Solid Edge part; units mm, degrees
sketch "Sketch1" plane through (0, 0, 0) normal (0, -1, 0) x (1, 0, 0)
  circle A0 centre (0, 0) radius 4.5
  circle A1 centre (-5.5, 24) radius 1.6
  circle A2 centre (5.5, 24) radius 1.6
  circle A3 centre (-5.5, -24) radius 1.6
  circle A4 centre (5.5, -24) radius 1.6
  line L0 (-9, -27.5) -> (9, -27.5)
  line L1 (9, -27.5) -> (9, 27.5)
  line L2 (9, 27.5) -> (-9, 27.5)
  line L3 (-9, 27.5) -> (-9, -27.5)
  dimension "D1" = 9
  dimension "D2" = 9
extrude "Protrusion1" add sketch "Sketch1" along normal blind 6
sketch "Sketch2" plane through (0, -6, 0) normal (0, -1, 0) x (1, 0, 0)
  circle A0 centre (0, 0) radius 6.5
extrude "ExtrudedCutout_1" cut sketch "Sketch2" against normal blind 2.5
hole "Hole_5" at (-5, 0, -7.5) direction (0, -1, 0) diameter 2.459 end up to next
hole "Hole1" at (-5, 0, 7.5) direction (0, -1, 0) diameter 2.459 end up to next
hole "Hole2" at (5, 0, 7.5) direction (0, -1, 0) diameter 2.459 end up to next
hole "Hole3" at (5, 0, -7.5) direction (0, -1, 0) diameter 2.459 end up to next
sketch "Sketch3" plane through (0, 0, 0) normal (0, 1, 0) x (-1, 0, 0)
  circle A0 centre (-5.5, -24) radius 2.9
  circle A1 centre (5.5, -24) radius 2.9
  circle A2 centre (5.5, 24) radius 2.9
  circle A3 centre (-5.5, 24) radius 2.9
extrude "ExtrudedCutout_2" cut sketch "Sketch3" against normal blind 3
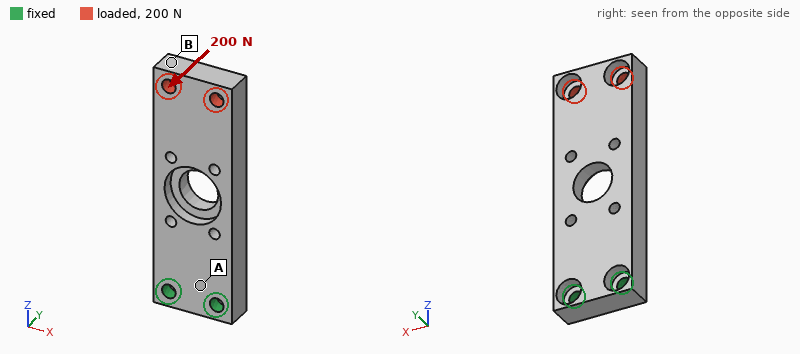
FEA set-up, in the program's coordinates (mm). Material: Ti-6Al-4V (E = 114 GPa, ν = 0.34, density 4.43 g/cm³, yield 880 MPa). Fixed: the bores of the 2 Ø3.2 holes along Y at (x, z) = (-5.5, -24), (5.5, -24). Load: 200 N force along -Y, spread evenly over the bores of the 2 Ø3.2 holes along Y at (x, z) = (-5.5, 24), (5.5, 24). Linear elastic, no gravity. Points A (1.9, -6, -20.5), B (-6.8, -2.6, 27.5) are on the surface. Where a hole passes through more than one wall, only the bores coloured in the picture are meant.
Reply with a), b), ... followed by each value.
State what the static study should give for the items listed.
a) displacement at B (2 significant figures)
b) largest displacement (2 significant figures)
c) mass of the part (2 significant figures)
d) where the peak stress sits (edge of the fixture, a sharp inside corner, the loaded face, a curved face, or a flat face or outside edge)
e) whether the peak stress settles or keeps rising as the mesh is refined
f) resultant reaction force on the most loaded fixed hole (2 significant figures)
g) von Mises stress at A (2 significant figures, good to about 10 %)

a) 0.42 mm
b) 0.42 mm
c) 22 g
d) edge of the fixture
e) keeps rising
f) 130 N
g) 92 MPa
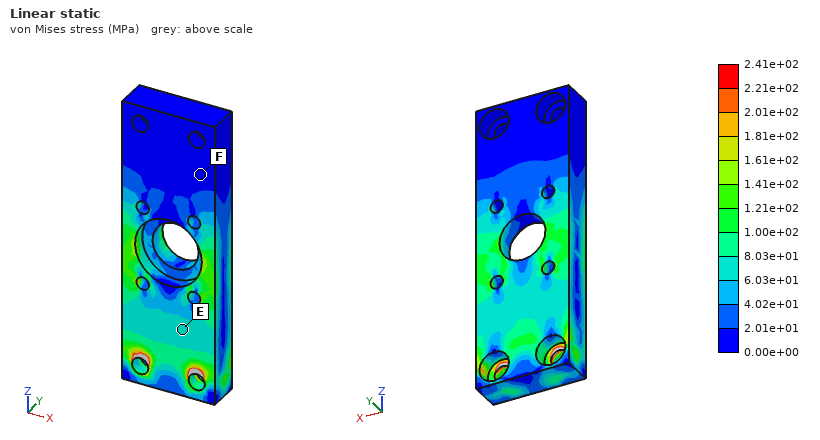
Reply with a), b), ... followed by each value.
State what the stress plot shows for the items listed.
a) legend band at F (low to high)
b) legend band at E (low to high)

a) 0.00e+00 to 2.01e+01 MPa
b) 6.03e+01 to 8.03e+01 MPa
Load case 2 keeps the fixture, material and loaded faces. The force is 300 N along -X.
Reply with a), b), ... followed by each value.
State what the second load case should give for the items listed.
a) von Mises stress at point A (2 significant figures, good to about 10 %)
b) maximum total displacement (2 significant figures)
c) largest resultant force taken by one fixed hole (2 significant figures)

a) 30 MPa
b) 66 µm
c) 1.1 kN
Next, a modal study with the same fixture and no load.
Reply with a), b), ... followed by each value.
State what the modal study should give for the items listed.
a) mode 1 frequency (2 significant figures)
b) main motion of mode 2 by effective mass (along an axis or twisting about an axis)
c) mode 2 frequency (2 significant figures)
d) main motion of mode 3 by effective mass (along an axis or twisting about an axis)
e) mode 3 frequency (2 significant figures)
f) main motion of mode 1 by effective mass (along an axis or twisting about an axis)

a) 1500 Hz
b) along X
c) 4500 Hz
d) twisting about Z
e) 7600 Hz
f) along Y
